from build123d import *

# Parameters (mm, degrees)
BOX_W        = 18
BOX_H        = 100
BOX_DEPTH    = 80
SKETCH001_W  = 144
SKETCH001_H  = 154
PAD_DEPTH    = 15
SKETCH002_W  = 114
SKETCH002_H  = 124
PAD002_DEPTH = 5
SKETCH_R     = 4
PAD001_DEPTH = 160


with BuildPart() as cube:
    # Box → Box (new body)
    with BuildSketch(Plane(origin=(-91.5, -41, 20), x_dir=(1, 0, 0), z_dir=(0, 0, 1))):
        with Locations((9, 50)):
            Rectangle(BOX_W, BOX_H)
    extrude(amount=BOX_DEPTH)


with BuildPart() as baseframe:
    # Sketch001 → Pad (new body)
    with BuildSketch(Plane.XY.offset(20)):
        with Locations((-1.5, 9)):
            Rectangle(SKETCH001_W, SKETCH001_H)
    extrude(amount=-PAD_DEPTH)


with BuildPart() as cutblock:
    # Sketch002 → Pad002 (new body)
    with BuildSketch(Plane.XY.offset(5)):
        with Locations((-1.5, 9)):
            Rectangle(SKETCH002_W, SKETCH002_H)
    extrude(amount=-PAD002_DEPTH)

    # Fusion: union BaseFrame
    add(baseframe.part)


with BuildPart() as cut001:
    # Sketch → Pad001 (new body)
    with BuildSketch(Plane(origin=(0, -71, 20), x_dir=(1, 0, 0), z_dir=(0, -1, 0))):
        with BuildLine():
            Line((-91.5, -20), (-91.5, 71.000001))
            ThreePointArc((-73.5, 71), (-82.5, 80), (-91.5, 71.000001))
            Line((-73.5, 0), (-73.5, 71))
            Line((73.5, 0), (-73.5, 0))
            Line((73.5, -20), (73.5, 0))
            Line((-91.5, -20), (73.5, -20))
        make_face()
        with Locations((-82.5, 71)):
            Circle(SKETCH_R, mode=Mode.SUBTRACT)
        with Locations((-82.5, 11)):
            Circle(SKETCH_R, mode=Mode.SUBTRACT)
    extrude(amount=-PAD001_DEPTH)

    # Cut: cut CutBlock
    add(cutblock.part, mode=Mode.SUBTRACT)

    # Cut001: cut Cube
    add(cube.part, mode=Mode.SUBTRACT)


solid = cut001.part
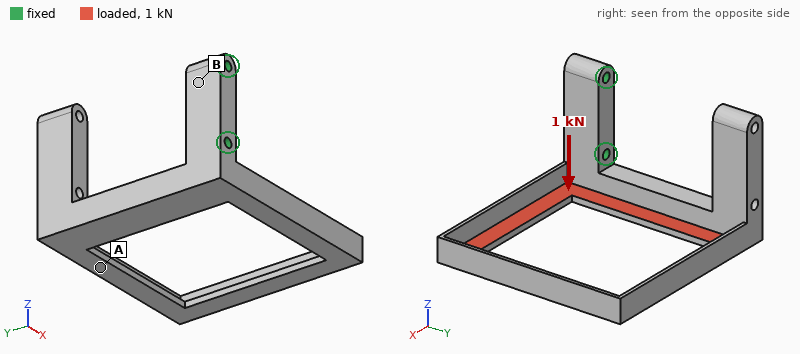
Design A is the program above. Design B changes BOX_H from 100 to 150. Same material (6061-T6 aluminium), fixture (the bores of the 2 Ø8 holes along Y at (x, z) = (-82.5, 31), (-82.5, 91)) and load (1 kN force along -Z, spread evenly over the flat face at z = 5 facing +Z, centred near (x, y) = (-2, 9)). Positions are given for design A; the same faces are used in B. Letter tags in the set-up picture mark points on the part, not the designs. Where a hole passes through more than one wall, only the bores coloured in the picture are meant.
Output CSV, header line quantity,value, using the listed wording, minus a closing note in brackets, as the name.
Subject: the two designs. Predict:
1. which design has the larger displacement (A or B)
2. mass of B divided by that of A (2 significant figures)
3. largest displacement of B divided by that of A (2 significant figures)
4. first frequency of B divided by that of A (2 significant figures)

quantity,value
which design has the larger displacement,B
mass of B divided by that of A,0.68
largest displacement of B divided by that of A,5.1
first frequency of B divided by that of A,0.37
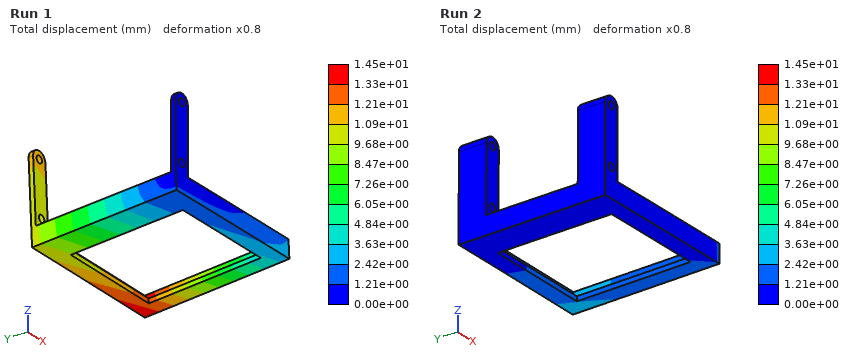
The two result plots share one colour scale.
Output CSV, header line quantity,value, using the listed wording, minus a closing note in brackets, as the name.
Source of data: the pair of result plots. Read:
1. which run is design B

quantity,value
which run is design B,Run 1
